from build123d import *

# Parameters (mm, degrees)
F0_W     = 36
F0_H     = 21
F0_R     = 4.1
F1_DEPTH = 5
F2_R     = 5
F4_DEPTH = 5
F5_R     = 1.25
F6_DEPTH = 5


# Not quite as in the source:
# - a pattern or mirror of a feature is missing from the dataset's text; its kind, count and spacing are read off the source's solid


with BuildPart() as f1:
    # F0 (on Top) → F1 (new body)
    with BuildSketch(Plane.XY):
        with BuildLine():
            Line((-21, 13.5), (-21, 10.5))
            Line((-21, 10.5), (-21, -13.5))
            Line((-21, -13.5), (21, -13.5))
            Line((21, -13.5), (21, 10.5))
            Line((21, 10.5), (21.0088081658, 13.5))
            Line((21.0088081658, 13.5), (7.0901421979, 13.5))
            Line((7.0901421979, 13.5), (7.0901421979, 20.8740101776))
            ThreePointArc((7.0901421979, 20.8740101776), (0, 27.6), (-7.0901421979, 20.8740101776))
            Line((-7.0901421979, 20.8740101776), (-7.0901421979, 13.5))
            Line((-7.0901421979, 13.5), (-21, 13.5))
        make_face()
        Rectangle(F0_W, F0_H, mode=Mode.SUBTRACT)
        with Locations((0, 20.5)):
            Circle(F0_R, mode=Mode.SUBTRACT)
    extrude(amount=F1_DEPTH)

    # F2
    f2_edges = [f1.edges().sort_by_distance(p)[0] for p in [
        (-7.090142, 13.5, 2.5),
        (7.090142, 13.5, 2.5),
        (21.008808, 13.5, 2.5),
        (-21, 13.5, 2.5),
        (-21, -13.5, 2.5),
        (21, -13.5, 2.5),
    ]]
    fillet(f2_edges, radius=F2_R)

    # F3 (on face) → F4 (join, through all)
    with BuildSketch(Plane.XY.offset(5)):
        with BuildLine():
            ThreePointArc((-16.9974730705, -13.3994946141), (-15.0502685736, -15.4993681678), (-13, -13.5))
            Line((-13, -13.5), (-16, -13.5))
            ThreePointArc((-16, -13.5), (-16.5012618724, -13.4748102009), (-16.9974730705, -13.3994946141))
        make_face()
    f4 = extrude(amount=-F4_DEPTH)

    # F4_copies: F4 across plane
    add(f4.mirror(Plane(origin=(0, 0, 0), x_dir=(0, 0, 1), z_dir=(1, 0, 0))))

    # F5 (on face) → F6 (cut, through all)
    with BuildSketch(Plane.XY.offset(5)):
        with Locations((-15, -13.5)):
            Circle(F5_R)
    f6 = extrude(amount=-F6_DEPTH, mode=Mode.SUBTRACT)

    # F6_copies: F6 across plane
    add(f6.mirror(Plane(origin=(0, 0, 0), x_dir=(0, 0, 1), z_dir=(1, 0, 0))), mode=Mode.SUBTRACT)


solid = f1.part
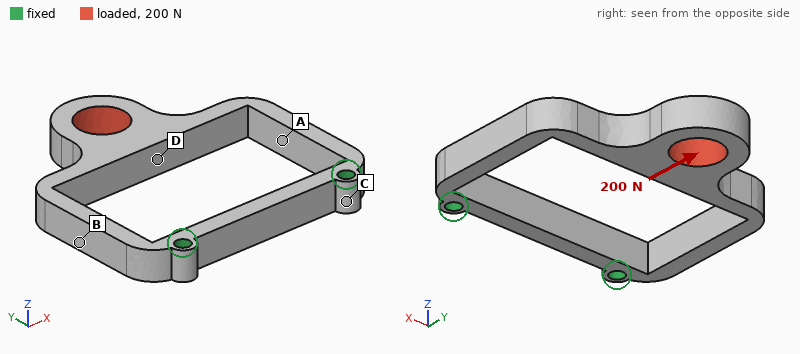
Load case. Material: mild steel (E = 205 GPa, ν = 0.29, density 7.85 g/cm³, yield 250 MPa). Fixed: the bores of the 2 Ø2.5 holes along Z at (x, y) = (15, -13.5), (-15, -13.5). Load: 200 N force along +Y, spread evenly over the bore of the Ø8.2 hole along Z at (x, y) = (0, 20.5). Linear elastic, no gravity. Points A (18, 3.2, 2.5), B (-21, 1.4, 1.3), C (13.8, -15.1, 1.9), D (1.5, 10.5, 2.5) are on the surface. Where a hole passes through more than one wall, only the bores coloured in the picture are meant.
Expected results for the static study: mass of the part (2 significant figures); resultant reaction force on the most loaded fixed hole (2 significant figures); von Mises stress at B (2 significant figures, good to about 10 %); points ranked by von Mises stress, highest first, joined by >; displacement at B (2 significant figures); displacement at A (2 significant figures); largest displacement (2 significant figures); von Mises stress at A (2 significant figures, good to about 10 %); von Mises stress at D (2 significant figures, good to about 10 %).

19 g
100 N
17 MPa
A > D > B > C
6.0 µm
6.0 µm
17 µm
34 MPa
25 MPa
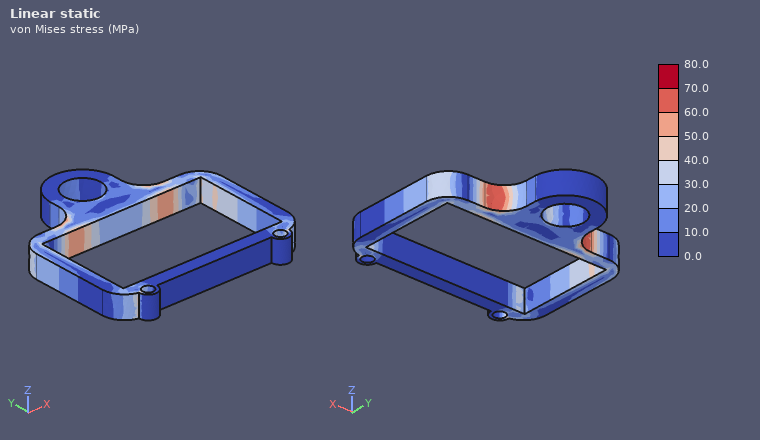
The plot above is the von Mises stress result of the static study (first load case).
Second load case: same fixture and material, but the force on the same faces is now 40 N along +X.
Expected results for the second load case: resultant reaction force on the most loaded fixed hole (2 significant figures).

30 N
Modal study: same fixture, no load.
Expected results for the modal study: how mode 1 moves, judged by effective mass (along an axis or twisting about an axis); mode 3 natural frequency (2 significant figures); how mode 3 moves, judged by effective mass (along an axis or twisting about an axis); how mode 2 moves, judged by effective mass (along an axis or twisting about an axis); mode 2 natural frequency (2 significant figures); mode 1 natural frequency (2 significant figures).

along Z
4700 Hz
twisting about Y
along X
1800 Hz
1400 Hz
